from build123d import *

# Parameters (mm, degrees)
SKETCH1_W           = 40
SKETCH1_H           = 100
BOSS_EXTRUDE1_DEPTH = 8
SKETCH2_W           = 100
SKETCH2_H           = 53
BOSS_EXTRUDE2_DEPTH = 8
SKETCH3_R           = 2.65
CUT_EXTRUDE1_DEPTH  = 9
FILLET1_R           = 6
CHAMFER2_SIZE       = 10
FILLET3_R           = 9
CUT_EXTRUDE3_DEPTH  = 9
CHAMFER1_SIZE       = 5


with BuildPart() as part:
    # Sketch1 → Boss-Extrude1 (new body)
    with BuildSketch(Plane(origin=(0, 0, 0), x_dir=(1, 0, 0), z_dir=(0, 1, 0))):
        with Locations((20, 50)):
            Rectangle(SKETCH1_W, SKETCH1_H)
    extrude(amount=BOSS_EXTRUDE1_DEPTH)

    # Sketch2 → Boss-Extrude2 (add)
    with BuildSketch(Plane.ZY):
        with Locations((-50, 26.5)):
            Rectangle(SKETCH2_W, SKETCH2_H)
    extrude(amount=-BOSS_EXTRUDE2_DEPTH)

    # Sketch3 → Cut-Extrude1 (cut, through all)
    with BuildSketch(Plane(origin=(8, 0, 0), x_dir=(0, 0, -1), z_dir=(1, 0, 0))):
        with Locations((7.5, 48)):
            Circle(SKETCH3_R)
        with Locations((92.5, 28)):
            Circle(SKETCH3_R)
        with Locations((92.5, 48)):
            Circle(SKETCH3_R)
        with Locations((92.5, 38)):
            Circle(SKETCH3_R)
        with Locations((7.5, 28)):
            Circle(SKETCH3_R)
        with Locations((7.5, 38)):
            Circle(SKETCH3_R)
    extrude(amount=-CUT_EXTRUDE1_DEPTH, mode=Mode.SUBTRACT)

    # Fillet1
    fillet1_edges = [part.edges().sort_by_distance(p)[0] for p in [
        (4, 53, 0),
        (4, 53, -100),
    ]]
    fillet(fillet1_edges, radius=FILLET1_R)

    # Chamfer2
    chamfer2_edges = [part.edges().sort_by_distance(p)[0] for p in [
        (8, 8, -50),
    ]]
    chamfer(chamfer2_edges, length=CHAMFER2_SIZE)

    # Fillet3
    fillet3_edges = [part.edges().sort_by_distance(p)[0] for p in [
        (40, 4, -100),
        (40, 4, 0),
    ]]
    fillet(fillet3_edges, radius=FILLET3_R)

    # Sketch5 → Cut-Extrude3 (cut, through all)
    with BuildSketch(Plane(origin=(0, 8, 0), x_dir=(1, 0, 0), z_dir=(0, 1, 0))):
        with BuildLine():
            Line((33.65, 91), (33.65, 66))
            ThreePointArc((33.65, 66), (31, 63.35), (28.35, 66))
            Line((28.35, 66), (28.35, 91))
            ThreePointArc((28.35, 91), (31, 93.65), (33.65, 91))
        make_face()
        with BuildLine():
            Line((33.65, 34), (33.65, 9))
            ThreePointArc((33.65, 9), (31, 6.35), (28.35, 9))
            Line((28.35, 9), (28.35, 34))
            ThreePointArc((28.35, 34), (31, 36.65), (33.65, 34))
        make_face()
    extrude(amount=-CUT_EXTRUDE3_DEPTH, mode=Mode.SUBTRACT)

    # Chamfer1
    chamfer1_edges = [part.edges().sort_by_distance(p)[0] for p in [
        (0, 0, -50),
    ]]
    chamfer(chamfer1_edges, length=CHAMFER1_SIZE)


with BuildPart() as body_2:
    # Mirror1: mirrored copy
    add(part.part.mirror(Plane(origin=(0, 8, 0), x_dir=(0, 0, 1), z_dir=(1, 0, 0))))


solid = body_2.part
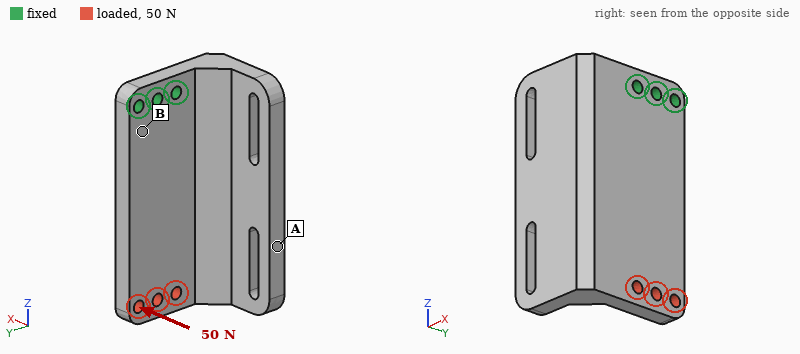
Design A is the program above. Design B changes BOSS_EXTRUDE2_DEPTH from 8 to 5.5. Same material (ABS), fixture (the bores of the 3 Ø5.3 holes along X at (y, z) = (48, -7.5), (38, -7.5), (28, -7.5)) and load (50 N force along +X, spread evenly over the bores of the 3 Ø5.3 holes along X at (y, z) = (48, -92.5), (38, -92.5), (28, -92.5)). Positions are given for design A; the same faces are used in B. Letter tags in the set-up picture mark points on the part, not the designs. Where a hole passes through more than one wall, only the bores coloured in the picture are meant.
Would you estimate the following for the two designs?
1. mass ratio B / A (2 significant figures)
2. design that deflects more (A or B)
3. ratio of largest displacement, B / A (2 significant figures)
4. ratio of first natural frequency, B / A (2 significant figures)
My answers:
0.84
B
2.4
0.68
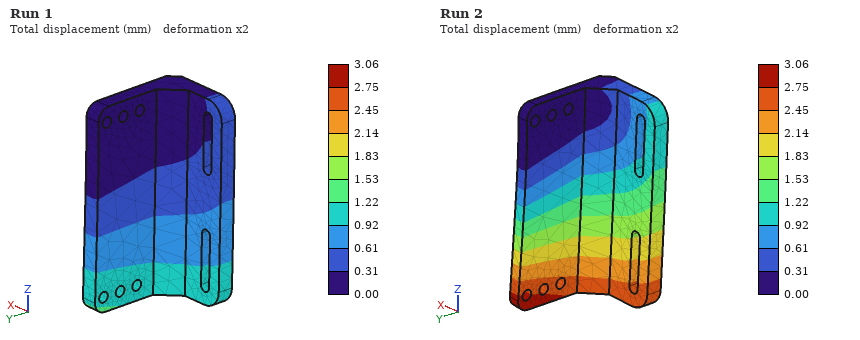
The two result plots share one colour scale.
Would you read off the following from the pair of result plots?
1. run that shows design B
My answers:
Run 2
